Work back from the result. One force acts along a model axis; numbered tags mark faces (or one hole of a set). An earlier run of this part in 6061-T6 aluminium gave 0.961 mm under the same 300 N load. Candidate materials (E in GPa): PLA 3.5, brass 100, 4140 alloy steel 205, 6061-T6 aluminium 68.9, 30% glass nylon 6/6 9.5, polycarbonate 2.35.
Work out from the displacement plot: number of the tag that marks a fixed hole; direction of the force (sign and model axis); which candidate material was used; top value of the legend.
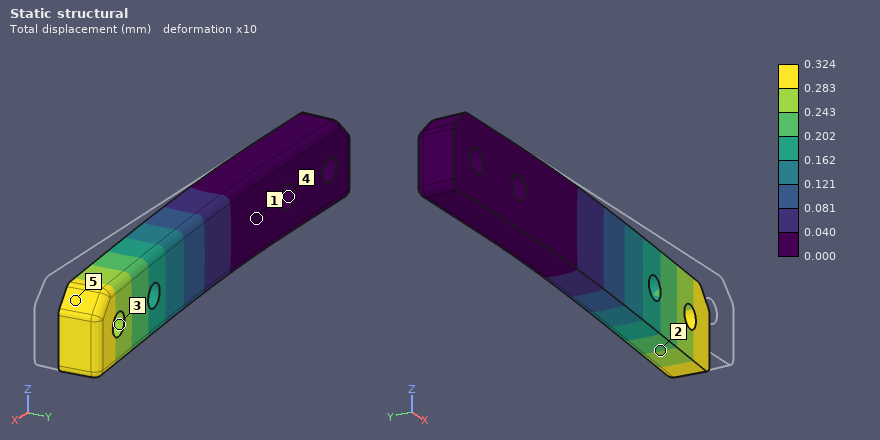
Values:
4
+Y
4140 alloy steel
0.324 mm
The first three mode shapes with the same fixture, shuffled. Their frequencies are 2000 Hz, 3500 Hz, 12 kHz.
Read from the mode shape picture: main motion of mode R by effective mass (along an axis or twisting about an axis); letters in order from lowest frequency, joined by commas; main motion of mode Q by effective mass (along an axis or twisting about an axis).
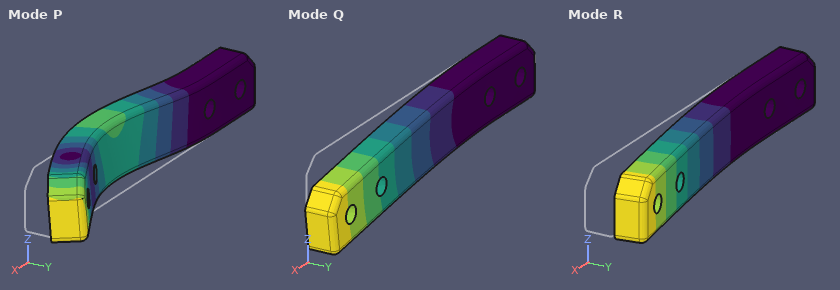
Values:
along Y
R, Q, P
along Z
